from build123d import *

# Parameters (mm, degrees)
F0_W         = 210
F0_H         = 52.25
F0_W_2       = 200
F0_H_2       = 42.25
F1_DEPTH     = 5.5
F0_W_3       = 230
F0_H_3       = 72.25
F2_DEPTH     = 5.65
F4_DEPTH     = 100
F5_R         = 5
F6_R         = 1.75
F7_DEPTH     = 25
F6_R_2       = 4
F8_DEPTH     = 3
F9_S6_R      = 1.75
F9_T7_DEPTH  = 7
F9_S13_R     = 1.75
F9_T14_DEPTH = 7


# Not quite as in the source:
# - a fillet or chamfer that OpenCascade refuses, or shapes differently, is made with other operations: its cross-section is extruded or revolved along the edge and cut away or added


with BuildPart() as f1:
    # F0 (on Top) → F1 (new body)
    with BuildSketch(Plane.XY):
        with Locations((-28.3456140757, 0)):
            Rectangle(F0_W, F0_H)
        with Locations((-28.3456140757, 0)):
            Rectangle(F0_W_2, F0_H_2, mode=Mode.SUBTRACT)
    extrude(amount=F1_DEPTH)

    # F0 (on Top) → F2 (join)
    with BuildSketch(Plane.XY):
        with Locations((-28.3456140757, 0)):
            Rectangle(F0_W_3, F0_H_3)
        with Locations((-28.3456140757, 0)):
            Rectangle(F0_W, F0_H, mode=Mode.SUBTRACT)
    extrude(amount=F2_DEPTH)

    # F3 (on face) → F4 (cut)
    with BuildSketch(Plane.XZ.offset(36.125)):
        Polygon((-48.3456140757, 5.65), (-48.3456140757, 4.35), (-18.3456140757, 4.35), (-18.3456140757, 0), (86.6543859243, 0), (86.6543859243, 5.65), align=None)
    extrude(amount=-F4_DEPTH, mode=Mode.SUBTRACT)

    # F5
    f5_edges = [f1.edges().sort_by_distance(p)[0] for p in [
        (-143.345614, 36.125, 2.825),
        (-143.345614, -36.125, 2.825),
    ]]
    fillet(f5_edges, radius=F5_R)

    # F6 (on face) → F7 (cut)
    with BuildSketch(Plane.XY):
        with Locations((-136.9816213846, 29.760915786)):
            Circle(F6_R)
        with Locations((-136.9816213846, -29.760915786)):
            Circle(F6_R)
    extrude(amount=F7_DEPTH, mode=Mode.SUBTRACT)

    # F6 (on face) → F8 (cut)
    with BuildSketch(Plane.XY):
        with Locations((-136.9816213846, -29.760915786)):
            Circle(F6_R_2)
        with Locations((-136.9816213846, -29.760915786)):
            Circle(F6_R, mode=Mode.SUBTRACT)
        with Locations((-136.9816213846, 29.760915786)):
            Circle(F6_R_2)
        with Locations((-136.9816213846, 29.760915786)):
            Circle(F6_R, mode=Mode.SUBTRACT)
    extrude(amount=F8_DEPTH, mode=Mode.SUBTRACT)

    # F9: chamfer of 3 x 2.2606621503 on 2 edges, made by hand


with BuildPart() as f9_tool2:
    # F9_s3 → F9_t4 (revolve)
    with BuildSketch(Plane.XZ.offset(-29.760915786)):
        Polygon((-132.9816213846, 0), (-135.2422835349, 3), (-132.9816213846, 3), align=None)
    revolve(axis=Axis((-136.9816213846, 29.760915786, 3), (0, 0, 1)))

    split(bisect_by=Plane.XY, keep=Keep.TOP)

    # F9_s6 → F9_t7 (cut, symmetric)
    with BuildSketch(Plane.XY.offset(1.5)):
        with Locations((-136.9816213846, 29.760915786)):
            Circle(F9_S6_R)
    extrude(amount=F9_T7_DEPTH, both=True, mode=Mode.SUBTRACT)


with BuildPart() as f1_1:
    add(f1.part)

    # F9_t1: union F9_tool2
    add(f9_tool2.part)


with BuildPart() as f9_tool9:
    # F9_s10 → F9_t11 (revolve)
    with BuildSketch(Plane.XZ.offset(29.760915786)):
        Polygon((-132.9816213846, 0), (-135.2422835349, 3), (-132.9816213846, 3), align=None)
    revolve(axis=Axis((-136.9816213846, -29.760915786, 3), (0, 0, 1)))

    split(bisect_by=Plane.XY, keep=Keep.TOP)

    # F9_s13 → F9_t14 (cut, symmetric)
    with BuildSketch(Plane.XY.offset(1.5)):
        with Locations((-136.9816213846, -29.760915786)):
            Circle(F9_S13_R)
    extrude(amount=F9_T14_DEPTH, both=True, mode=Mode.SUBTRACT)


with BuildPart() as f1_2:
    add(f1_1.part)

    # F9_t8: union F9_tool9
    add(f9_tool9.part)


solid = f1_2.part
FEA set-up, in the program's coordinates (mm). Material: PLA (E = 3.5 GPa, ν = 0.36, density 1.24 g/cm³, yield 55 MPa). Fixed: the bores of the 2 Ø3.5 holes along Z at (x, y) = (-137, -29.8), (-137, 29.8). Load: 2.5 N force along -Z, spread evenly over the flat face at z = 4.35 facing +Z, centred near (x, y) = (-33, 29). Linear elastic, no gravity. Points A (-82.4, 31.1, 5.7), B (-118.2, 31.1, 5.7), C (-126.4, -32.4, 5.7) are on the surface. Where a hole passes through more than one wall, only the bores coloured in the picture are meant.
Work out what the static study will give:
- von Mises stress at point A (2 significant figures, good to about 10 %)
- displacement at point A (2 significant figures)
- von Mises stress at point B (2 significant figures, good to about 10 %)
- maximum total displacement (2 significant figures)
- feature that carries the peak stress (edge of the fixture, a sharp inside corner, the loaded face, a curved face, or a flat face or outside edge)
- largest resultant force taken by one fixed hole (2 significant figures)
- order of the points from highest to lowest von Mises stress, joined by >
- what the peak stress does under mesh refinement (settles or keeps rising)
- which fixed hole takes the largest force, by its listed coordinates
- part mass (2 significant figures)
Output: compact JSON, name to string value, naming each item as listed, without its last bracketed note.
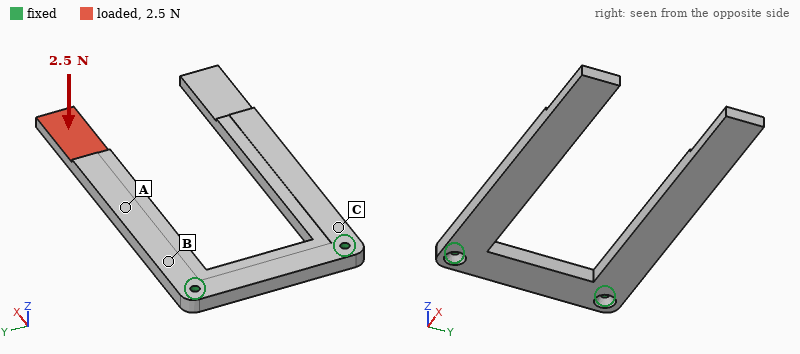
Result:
{"von Mises stress at point A": "1.6 MPa", "displacement at point A": "0.50 mm", "von Mises stress at point B": "2.7 MPa", "maximum total displacement": "1.7 mm", "feature that carries the peak stress": "edge of the fixture", "largest resultant force taken by one fixed hole": "2.9 N", "order of the points from highest to lowest von Mises stress, joined by >": "B > A > C", "what the peak stress does under mesh refinement": "keeps rising", "which fixed hole takes the largest force, by its listed coordinates": "(-137, 29.8)", "part mass": "29 g"}
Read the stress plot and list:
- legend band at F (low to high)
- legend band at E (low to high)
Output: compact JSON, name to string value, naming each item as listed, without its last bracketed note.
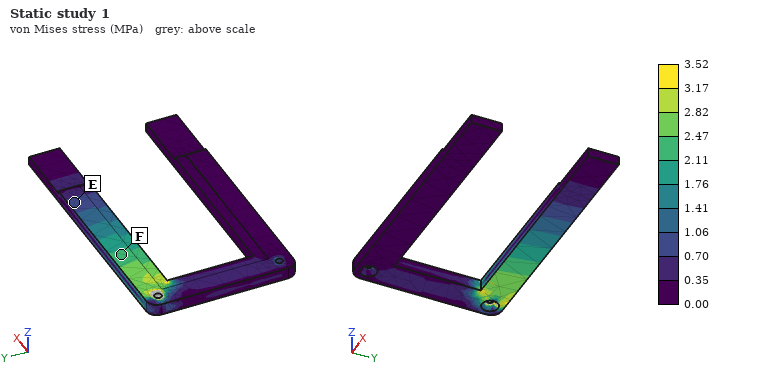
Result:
{"legend band at F": "2.11 to 2.47 MPa", "legend band at E": "0.70 to 1.06 MPa"}
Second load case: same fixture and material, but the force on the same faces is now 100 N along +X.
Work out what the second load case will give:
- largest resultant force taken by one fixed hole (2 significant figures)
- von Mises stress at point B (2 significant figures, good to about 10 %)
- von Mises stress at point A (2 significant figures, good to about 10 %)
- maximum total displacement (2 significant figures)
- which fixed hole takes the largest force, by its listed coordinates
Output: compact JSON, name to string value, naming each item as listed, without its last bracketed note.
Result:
{"largest resultant force taken by one fixed hole": "98 N", "von Mises stress at point B": "3.2 MPa", "von Mises stress at point A": "3.2 MPa", "maximum total displacement": "1.5 mm", "which fixed hole takes the largest force, by its listed coordinates": "(-137, 29.8)"}
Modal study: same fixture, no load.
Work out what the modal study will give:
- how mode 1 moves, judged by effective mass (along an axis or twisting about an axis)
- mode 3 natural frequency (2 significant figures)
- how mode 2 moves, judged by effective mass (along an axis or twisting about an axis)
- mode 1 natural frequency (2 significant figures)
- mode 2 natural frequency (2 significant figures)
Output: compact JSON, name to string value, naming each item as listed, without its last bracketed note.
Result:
{"how mode 1 moves, judged by effective mass": "along Z", "mode 3 natural frequency": "260 Hz", "how mode 2 moves, judged by effective mass": "twisting about X", "mode 1 natural frequency": "110 Hz", "mode 2 natural frequency": "110 Hz"}
